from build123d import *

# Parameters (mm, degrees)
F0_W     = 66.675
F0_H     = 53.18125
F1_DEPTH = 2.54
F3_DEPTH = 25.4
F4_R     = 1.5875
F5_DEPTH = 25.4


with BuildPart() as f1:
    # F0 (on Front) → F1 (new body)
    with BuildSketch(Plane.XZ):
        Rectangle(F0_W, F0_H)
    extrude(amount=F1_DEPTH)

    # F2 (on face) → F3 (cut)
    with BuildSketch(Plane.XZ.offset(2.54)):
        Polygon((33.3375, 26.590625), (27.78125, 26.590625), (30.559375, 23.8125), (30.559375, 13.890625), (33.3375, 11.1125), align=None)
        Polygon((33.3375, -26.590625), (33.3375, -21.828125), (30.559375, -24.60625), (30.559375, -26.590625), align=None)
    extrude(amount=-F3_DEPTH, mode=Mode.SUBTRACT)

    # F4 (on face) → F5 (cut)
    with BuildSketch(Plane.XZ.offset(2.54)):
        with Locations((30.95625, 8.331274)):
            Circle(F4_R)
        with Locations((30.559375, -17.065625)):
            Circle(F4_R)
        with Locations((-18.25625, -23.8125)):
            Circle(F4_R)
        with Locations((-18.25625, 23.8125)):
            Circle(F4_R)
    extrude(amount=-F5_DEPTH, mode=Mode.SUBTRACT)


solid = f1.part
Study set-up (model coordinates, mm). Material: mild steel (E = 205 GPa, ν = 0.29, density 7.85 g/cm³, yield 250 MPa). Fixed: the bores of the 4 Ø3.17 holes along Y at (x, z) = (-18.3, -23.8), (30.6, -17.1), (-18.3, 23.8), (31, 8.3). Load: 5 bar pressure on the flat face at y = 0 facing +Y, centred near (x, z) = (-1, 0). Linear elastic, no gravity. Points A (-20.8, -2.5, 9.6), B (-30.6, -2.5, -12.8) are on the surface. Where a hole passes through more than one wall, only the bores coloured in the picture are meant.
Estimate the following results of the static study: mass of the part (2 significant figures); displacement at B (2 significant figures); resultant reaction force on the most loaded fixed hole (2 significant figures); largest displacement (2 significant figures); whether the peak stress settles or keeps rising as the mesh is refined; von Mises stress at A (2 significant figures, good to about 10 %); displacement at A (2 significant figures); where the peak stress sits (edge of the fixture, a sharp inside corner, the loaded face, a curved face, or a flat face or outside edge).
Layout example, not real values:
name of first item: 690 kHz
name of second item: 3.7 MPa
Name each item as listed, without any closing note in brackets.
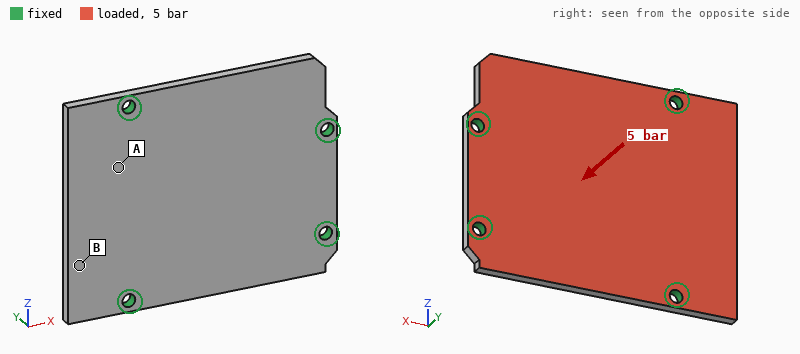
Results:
mass of the part: 69 g
displacement at B: 25 µm
resultant reaction force on the most loaded fixed hole: 530 N
largest displacement: 49 µm
whether the peak stress settles or keeps rising as the mesh is refined: keeps rising
von Mises stress at A: 47 MPa
displacement at A: 27 µm
where the peak stress sits: edge of the fixture
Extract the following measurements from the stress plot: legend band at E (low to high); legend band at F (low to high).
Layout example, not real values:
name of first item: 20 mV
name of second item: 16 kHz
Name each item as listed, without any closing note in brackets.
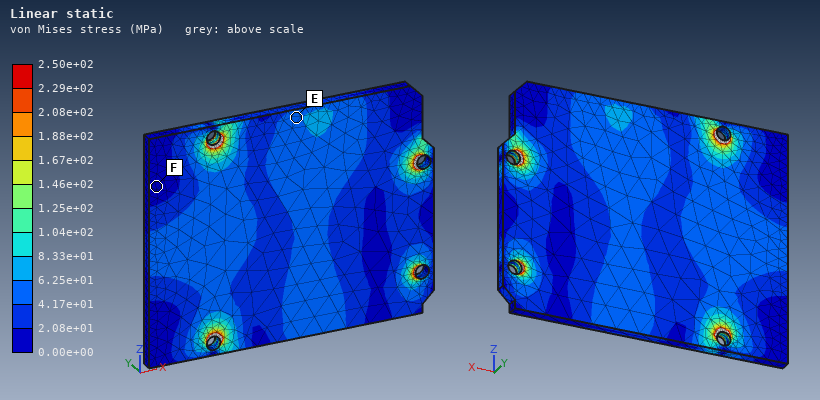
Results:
legend band at E: 4.17e+01 to 6.25e+01 MPa
legend band at F: 0.00e+00 to 2.08e+01 MPa
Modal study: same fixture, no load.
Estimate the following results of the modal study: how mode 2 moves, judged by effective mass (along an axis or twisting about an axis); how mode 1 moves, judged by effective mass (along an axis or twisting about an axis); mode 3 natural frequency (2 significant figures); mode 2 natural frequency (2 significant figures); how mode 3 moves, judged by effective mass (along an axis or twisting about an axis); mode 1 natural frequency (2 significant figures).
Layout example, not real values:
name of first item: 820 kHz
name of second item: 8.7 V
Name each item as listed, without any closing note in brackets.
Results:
how mode 2 moves, judged by effective mass: along Y
how mode 1 moves, judged by effective mass: along Y
mode 3 natural frequency: 5200 Hz
mode 2 natural frequency: 4700 Hz
how mode 3 moves, judged by effective mass: twisting about X
mode 1 natural frequency: 4200 Hz
